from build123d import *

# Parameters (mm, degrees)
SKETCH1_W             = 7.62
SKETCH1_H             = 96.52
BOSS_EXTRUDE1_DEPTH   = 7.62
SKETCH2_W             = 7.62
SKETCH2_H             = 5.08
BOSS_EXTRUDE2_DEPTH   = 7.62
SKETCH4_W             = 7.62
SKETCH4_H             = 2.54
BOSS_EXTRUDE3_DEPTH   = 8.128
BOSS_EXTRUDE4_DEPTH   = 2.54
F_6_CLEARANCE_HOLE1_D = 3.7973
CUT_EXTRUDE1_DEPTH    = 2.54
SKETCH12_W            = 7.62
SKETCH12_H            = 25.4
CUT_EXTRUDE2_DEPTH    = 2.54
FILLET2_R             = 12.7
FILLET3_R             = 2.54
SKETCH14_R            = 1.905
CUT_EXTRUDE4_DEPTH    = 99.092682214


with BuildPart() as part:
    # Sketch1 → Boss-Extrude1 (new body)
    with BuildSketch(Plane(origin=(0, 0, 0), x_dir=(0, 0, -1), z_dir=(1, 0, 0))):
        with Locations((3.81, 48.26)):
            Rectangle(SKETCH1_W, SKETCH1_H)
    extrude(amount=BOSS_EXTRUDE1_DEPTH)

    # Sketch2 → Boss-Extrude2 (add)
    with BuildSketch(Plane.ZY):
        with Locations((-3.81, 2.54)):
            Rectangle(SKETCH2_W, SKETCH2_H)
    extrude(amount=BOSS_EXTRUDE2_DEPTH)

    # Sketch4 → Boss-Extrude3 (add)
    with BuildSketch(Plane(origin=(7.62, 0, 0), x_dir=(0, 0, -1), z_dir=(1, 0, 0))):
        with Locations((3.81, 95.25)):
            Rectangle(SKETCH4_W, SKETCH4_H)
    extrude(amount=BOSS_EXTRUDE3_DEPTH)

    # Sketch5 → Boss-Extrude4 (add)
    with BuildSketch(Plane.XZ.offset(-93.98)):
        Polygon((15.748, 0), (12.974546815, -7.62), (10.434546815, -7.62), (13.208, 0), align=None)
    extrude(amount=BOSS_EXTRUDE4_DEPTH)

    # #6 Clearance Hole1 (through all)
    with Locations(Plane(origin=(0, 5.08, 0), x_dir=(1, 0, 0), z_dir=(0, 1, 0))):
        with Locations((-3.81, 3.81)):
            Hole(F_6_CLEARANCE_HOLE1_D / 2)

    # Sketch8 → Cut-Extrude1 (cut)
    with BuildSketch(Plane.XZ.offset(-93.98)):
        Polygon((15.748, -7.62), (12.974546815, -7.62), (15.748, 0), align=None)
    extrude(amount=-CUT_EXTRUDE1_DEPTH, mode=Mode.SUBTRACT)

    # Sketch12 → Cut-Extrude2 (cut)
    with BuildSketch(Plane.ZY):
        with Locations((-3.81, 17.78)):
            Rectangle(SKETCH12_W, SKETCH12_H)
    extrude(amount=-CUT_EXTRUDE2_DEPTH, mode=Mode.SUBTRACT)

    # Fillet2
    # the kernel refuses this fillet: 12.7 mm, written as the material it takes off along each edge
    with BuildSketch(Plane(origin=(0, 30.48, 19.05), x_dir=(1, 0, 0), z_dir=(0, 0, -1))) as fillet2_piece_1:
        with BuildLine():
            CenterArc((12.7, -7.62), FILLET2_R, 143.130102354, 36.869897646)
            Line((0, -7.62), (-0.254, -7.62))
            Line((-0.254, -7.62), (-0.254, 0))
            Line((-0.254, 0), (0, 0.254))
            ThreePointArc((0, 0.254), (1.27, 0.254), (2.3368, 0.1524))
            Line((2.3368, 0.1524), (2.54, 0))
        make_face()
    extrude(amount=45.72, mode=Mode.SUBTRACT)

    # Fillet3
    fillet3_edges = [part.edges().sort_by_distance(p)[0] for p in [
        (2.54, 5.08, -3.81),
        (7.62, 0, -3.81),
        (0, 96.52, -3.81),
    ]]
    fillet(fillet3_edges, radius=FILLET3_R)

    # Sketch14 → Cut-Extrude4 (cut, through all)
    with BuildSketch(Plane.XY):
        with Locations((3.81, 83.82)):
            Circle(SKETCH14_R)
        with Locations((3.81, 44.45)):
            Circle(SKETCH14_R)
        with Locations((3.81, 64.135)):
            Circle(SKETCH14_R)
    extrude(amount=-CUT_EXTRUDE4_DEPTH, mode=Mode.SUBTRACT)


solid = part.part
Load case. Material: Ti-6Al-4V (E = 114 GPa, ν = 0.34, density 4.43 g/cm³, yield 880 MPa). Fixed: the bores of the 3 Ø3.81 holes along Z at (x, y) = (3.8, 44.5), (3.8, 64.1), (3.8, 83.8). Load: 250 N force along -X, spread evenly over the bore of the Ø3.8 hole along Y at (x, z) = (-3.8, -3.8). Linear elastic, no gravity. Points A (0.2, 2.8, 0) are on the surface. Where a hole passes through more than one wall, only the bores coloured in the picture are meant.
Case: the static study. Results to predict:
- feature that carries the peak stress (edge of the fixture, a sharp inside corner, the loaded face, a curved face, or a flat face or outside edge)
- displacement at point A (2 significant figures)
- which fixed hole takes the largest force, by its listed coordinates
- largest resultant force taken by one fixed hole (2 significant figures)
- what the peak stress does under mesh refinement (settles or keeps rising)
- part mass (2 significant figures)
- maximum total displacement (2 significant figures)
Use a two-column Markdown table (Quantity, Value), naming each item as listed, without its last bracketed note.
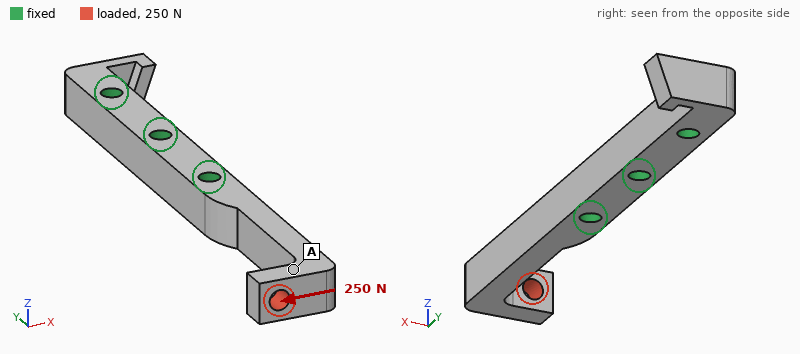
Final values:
| Quantity | Value |
|---|---|
| feature that carries the peak stress | a sharp inside corner |
| displacement at point A | 0.38 mm |
| which fixed hole takes the largest force, by its listed coordinates | (3.8, 44.5) |
| largest resultant force taken by one fixed hole | 340 N |
| what the peak stress does under mesh refinement | keeps rising |
| part mass | 23 g |
| maximum total displacement | 0.46 mm |
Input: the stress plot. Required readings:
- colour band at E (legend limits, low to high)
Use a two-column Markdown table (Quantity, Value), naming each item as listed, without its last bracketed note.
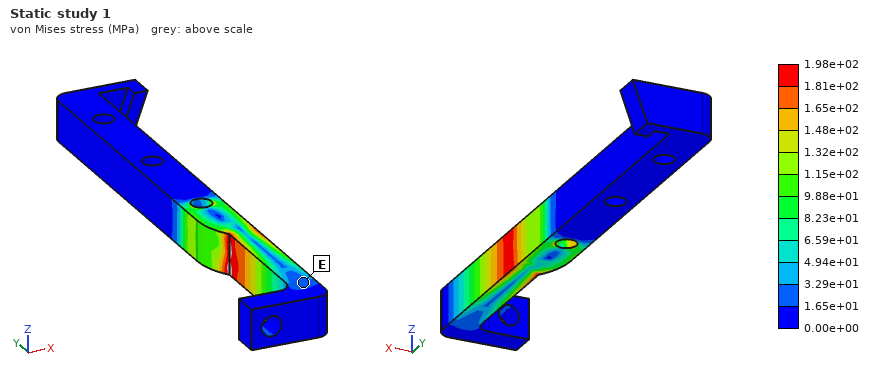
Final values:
| Quantity | Value |
|---|---|
| colour band at E | 1.65e+01 to 3.29e+01 MPa |
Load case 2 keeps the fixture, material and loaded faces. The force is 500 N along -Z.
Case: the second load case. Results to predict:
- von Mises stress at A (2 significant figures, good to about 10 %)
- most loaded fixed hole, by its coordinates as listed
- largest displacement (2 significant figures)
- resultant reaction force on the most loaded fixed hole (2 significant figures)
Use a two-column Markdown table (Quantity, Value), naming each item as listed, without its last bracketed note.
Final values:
| Quantity | Value |
|---|---|
| von Mises stress at A | 45 MPa |
| most loaded fixed hole, by its coordinates as listed | (3.8, 44.5) |
| largest displacement | 0.73 mm |
| resultant reaction force on the most loaded fixed hole | 550 N |
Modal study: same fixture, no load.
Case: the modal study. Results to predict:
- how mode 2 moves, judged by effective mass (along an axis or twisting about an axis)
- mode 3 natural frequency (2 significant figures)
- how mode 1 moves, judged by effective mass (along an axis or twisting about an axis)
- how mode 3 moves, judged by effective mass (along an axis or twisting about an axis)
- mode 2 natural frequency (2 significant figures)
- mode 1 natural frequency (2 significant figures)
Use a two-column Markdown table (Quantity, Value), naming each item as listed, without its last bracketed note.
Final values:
| Quantity | Value |
|---|---|
| how mode 2 moves, judged by effective mass | along Z |
| mode 3 natural frequency | 8600 Hz |
| how mode 1 moves, judged by effective mass | along X |
| how mode 3 moves, judged by effective mass | twisting about Y |
| mode 2 natural frequency | 2700 Hz |
| mode 1 natural frequency | 2200 Hz |
